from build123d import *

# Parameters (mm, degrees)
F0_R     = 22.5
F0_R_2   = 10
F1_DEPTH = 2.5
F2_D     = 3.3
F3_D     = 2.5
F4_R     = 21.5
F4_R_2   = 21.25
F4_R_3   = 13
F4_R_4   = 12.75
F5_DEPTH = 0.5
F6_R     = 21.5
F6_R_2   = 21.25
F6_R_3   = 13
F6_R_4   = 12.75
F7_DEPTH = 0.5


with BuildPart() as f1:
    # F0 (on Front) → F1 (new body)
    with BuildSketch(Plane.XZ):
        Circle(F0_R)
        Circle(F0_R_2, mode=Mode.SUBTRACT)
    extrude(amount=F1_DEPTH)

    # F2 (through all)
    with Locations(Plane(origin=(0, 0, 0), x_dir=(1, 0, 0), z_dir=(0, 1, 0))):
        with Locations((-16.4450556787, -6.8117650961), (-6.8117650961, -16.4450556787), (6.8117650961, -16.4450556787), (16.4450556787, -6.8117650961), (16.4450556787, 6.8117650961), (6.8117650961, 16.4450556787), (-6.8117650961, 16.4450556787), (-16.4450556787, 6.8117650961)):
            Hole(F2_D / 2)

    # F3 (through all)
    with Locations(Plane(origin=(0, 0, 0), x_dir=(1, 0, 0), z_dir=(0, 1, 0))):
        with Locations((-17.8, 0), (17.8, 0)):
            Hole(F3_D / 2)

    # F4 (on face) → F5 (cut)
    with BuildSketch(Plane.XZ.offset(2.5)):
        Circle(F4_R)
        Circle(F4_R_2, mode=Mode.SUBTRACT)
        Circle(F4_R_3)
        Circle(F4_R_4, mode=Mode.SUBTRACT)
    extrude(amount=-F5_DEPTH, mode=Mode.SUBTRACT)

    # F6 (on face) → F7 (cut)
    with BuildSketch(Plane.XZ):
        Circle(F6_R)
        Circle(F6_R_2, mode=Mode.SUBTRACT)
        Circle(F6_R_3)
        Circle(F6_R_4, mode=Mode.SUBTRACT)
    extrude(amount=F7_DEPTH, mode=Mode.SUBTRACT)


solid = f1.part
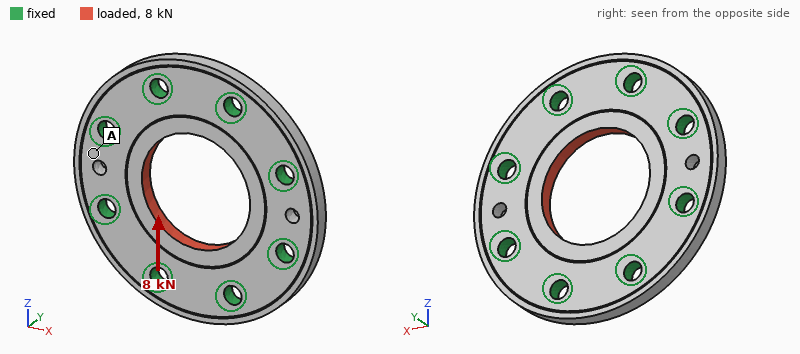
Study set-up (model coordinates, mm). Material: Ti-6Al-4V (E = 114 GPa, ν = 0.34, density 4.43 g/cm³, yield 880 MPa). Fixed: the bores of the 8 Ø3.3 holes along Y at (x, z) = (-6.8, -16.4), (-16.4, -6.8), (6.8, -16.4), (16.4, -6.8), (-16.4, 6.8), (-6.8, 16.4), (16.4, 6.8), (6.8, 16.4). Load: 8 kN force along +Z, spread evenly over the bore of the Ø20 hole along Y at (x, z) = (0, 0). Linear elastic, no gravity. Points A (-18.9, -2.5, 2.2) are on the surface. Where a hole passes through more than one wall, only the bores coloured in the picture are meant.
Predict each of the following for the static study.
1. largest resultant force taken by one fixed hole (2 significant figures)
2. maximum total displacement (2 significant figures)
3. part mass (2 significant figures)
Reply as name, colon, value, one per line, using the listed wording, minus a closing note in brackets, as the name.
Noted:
largest resultant force taken by one fixed hole: 1.4 kN
maximum total displacement: 5.1 µm
part mass: 13 g
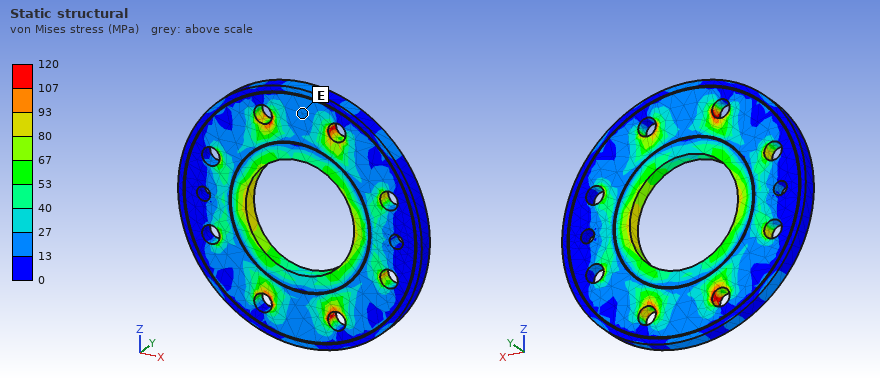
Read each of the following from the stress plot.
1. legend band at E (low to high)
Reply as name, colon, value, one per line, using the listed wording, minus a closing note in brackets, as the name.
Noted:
legend band at E: 13 to 27 MPa
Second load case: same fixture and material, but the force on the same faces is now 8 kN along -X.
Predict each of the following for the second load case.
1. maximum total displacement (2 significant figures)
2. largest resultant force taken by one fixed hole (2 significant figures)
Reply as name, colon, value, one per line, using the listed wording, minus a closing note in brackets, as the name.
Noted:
maximum total displacement: 5.1 µm
largest resultant force taken by one fixed hole: 1.4 kN
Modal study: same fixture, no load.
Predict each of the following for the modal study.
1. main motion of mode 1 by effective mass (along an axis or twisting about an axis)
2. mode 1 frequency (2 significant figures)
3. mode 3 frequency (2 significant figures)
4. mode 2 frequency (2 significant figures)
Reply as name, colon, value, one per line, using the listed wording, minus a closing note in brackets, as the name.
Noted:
main motion of mode 1 by effective mass: along Y
mode 1 frequency: 39 kHz
mode 3 frequency: 43 kHz
mode 2 frequency: 43 kHz
